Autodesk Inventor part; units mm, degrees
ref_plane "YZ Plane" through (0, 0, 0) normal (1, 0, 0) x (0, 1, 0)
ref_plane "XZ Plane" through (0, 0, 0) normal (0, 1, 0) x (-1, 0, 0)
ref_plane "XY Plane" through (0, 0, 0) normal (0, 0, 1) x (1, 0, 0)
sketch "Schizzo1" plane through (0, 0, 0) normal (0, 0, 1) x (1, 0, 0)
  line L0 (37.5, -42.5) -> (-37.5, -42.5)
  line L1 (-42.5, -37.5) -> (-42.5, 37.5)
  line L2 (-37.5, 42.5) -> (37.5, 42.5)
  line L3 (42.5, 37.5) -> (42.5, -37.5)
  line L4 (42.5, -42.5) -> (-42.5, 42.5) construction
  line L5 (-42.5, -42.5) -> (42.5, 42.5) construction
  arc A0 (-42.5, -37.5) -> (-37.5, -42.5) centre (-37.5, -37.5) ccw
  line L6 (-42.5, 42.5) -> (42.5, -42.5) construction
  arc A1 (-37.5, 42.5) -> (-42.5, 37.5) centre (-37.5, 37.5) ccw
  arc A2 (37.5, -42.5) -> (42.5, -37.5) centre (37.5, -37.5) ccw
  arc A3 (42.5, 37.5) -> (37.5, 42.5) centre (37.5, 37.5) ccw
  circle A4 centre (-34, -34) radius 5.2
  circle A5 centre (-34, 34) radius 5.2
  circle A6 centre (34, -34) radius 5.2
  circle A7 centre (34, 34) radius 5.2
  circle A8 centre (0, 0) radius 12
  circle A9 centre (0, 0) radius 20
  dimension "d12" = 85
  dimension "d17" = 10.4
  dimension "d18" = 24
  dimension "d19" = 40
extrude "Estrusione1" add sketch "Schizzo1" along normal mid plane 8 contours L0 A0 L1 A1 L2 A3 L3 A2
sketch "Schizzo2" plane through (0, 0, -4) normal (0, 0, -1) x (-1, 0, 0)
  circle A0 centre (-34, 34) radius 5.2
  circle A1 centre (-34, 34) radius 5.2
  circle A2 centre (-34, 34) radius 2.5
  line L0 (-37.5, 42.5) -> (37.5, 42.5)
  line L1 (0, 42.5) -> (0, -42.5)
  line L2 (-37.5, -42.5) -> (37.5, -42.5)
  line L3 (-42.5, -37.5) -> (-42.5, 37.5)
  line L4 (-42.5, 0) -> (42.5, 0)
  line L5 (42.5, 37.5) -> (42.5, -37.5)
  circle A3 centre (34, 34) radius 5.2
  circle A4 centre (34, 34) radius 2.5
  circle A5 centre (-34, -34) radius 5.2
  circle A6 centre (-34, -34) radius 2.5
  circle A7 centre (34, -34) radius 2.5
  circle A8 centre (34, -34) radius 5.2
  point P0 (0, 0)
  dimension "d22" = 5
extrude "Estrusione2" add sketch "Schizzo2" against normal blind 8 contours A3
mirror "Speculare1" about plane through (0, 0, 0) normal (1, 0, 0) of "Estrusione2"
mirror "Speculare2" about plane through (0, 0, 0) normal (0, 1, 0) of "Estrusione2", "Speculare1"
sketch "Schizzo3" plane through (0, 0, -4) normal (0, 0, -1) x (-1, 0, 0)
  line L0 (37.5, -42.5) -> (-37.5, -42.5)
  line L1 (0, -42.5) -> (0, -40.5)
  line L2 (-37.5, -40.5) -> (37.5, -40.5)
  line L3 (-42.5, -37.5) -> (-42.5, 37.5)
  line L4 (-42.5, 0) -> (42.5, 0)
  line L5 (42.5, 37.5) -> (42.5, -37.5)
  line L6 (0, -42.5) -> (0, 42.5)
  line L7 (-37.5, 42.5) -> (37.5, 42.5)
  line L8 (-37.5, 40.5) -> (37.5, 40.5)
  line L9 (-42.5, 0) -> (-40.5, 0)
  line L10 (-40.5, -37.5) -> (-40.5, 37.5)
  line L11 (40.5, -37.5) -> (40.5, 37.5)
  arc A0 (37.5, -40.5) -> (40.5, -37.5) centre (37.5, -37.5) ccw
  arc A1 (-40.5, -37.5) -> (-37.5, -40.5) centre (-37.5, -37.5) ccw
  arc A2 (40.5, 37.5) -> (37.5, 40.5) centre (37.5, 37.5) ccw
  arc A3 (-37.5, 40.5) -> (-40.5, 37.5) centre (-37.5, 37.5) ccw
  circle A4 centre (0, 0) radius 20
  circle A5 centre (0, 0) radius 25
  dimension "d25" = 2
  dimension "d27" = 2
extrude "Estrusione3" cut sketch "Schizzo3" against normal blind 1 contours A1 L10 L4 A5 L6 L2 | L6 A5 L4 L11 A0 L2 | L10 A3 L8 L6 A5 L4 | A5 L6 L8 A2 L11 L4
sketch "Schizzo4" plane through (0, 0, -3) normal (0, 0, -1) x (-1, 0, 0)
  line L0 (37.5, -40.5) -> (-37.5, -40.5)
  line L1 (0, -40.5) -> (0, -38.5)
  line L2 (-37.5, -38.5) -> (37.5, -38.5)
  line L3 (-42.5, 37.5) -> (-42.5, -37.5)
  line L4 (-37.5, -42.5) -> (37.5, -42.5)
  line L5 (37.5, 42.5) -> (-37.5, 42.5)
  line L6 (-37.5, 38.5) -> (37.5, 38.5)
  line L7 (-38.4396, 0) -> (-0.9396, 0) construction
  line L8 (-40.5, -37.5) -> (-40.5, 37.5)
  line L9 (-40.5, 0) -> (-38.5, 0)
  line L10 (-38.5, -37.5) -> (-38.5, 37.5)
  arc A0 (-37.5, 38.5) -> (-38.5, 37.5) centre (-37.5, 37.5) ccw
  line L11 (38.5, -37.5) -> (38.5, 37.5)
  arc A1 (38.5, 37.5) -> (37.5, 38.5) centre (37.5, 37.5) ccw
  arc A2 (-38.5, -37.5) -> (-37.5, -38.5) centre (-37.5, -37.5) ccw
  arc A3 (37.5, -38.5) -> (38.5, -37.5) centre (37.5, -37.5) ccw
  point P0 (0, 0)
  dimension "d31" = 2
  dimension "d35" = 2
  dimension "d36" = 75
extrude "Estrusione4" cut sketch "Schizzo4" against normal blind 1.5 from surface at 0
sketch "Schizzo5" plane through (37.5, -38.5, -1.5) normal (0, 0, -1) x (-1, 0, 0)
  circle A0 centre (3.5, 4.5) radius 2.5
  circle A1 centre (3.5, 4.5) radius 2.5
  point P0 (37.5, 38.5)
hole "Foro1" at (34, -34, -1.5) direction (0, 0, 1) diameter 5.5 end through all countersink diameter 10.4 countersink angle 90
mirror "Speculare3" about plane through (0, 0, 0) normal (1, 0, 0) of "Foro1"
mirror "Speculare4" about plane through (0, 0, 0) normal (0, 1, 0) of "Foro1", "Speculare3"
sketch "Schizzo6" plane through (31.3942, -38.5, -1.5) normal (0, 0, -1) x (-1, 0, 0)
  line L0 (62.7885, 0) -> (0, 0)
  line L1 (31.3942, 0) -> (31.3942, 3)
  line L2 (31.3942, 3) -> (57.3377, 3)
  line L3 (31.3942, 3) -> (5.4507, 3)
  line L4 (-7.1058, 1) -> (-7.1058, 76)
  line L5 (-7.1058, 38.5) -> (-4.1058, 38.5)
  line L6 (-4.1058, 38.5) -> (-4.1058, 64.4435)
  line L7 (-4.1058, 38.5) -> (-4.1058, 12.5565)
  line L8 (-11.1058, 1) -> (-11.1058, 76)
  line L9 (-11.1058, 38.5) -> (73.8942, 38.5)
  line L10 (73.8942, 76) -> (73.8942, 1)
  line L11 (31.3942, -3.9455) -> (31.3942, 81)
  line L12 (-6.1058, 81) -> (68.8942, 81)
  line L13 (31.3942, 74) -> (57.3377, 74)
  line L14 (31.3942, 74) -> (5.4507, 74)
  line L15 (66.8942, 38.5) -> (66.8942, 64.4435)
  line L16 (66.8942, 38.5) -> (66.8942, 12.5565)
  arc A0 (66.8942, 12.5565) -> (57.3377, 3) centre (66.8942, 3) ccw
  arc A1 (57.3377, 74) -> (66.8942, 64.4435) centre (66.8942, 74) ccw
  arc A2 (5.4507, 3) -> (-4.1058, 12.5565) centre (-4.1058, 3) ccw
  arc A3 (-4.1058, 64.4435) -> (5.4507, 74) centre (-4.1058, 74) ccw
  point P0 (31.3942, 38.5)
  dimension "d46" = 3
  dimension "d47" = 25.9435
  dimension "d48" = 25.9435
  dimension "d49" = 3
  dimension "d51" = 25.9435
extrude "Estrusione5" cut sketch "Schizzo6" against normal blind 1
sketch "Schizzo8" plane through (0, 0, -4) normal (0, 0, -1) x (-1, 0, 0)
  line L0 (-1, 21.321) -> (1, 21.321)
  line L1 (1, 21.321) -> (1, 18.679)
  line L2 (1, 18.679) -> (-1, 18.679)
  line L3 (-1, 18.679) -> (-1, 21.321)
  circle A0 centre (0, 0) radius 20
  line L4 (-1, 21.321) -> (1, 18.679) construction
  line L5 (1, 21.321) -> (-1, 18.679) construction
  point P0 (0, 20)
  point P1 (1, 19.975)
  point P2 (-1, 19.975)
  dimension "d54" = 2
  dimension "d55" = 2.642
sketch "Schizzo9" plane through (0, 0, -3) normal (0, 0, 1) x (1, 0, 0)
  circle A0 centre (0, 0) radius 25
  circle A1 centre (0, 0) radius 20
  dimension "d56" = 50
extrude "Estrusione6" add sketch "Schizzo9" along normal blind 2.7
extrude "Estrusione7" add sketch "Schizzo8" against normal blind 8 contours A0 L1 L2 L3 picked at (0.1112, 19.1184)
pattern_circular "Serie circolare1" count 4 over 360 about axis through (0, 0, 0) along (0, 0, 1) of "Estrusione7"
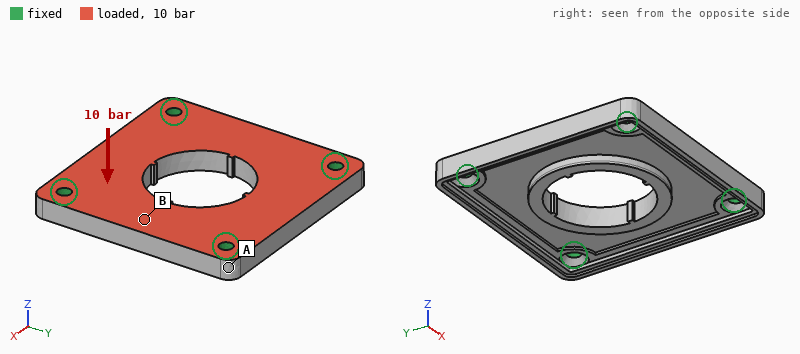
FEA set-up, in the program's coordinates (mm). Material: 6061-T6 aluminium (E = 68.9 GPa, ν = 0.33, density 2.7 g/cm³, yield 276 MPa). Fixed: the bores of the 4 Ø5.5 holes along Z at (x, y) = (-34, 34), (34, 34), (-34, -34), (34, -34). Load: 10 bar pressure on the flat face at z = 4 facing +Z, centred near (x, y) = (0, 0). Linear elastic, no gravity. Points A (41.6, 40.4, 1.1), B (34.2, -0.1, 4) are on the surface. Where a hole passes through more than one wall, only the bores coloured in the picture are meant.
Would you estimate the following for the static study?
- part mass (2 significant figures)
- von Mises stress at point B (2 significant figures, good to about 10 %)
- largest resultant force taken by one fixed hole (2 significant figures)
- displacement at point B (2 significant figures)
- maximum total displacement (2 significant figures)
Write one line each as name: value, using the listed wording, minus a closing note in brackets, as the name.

part mass: 91 g
von Mises stress at point B: 35 MPa
largest resultant force taken by one fixed hole: 1.7 kN
displacement at point B: 0.078 mm
maximum total displacement: 0.11 mm
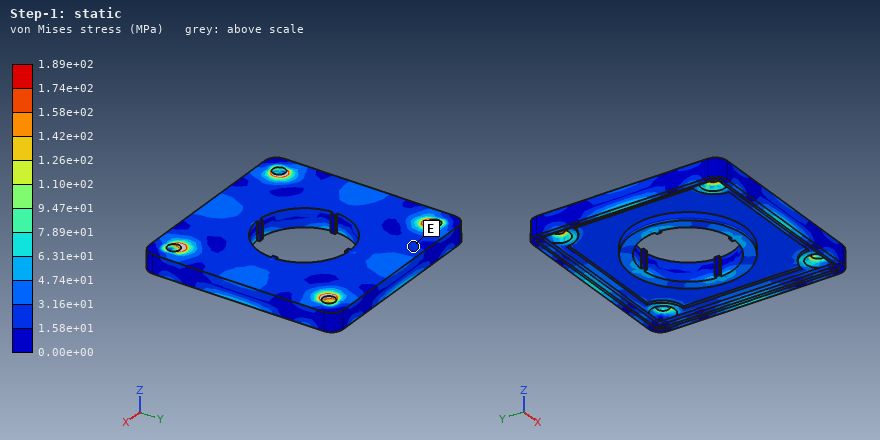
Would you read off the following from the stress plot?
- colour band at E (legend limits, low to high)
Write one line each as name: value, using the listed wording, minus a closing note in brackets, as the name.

colour band at E: 1.58e+01 to 3.16e+01 MPa
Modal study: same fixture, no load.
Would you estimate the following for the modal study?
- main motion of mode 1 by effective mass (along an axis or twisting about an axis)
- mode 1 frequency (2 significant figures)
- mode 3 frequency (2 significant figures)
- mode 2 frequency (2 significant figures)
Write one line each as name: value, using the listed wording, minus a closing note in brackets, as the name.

main motion of mode 1 by effective mass: along Z
mode 1 frequency: 4500 Hz
mode 3 frequency: 6000 Hz
mode 2 frequency: 6000 Hz
